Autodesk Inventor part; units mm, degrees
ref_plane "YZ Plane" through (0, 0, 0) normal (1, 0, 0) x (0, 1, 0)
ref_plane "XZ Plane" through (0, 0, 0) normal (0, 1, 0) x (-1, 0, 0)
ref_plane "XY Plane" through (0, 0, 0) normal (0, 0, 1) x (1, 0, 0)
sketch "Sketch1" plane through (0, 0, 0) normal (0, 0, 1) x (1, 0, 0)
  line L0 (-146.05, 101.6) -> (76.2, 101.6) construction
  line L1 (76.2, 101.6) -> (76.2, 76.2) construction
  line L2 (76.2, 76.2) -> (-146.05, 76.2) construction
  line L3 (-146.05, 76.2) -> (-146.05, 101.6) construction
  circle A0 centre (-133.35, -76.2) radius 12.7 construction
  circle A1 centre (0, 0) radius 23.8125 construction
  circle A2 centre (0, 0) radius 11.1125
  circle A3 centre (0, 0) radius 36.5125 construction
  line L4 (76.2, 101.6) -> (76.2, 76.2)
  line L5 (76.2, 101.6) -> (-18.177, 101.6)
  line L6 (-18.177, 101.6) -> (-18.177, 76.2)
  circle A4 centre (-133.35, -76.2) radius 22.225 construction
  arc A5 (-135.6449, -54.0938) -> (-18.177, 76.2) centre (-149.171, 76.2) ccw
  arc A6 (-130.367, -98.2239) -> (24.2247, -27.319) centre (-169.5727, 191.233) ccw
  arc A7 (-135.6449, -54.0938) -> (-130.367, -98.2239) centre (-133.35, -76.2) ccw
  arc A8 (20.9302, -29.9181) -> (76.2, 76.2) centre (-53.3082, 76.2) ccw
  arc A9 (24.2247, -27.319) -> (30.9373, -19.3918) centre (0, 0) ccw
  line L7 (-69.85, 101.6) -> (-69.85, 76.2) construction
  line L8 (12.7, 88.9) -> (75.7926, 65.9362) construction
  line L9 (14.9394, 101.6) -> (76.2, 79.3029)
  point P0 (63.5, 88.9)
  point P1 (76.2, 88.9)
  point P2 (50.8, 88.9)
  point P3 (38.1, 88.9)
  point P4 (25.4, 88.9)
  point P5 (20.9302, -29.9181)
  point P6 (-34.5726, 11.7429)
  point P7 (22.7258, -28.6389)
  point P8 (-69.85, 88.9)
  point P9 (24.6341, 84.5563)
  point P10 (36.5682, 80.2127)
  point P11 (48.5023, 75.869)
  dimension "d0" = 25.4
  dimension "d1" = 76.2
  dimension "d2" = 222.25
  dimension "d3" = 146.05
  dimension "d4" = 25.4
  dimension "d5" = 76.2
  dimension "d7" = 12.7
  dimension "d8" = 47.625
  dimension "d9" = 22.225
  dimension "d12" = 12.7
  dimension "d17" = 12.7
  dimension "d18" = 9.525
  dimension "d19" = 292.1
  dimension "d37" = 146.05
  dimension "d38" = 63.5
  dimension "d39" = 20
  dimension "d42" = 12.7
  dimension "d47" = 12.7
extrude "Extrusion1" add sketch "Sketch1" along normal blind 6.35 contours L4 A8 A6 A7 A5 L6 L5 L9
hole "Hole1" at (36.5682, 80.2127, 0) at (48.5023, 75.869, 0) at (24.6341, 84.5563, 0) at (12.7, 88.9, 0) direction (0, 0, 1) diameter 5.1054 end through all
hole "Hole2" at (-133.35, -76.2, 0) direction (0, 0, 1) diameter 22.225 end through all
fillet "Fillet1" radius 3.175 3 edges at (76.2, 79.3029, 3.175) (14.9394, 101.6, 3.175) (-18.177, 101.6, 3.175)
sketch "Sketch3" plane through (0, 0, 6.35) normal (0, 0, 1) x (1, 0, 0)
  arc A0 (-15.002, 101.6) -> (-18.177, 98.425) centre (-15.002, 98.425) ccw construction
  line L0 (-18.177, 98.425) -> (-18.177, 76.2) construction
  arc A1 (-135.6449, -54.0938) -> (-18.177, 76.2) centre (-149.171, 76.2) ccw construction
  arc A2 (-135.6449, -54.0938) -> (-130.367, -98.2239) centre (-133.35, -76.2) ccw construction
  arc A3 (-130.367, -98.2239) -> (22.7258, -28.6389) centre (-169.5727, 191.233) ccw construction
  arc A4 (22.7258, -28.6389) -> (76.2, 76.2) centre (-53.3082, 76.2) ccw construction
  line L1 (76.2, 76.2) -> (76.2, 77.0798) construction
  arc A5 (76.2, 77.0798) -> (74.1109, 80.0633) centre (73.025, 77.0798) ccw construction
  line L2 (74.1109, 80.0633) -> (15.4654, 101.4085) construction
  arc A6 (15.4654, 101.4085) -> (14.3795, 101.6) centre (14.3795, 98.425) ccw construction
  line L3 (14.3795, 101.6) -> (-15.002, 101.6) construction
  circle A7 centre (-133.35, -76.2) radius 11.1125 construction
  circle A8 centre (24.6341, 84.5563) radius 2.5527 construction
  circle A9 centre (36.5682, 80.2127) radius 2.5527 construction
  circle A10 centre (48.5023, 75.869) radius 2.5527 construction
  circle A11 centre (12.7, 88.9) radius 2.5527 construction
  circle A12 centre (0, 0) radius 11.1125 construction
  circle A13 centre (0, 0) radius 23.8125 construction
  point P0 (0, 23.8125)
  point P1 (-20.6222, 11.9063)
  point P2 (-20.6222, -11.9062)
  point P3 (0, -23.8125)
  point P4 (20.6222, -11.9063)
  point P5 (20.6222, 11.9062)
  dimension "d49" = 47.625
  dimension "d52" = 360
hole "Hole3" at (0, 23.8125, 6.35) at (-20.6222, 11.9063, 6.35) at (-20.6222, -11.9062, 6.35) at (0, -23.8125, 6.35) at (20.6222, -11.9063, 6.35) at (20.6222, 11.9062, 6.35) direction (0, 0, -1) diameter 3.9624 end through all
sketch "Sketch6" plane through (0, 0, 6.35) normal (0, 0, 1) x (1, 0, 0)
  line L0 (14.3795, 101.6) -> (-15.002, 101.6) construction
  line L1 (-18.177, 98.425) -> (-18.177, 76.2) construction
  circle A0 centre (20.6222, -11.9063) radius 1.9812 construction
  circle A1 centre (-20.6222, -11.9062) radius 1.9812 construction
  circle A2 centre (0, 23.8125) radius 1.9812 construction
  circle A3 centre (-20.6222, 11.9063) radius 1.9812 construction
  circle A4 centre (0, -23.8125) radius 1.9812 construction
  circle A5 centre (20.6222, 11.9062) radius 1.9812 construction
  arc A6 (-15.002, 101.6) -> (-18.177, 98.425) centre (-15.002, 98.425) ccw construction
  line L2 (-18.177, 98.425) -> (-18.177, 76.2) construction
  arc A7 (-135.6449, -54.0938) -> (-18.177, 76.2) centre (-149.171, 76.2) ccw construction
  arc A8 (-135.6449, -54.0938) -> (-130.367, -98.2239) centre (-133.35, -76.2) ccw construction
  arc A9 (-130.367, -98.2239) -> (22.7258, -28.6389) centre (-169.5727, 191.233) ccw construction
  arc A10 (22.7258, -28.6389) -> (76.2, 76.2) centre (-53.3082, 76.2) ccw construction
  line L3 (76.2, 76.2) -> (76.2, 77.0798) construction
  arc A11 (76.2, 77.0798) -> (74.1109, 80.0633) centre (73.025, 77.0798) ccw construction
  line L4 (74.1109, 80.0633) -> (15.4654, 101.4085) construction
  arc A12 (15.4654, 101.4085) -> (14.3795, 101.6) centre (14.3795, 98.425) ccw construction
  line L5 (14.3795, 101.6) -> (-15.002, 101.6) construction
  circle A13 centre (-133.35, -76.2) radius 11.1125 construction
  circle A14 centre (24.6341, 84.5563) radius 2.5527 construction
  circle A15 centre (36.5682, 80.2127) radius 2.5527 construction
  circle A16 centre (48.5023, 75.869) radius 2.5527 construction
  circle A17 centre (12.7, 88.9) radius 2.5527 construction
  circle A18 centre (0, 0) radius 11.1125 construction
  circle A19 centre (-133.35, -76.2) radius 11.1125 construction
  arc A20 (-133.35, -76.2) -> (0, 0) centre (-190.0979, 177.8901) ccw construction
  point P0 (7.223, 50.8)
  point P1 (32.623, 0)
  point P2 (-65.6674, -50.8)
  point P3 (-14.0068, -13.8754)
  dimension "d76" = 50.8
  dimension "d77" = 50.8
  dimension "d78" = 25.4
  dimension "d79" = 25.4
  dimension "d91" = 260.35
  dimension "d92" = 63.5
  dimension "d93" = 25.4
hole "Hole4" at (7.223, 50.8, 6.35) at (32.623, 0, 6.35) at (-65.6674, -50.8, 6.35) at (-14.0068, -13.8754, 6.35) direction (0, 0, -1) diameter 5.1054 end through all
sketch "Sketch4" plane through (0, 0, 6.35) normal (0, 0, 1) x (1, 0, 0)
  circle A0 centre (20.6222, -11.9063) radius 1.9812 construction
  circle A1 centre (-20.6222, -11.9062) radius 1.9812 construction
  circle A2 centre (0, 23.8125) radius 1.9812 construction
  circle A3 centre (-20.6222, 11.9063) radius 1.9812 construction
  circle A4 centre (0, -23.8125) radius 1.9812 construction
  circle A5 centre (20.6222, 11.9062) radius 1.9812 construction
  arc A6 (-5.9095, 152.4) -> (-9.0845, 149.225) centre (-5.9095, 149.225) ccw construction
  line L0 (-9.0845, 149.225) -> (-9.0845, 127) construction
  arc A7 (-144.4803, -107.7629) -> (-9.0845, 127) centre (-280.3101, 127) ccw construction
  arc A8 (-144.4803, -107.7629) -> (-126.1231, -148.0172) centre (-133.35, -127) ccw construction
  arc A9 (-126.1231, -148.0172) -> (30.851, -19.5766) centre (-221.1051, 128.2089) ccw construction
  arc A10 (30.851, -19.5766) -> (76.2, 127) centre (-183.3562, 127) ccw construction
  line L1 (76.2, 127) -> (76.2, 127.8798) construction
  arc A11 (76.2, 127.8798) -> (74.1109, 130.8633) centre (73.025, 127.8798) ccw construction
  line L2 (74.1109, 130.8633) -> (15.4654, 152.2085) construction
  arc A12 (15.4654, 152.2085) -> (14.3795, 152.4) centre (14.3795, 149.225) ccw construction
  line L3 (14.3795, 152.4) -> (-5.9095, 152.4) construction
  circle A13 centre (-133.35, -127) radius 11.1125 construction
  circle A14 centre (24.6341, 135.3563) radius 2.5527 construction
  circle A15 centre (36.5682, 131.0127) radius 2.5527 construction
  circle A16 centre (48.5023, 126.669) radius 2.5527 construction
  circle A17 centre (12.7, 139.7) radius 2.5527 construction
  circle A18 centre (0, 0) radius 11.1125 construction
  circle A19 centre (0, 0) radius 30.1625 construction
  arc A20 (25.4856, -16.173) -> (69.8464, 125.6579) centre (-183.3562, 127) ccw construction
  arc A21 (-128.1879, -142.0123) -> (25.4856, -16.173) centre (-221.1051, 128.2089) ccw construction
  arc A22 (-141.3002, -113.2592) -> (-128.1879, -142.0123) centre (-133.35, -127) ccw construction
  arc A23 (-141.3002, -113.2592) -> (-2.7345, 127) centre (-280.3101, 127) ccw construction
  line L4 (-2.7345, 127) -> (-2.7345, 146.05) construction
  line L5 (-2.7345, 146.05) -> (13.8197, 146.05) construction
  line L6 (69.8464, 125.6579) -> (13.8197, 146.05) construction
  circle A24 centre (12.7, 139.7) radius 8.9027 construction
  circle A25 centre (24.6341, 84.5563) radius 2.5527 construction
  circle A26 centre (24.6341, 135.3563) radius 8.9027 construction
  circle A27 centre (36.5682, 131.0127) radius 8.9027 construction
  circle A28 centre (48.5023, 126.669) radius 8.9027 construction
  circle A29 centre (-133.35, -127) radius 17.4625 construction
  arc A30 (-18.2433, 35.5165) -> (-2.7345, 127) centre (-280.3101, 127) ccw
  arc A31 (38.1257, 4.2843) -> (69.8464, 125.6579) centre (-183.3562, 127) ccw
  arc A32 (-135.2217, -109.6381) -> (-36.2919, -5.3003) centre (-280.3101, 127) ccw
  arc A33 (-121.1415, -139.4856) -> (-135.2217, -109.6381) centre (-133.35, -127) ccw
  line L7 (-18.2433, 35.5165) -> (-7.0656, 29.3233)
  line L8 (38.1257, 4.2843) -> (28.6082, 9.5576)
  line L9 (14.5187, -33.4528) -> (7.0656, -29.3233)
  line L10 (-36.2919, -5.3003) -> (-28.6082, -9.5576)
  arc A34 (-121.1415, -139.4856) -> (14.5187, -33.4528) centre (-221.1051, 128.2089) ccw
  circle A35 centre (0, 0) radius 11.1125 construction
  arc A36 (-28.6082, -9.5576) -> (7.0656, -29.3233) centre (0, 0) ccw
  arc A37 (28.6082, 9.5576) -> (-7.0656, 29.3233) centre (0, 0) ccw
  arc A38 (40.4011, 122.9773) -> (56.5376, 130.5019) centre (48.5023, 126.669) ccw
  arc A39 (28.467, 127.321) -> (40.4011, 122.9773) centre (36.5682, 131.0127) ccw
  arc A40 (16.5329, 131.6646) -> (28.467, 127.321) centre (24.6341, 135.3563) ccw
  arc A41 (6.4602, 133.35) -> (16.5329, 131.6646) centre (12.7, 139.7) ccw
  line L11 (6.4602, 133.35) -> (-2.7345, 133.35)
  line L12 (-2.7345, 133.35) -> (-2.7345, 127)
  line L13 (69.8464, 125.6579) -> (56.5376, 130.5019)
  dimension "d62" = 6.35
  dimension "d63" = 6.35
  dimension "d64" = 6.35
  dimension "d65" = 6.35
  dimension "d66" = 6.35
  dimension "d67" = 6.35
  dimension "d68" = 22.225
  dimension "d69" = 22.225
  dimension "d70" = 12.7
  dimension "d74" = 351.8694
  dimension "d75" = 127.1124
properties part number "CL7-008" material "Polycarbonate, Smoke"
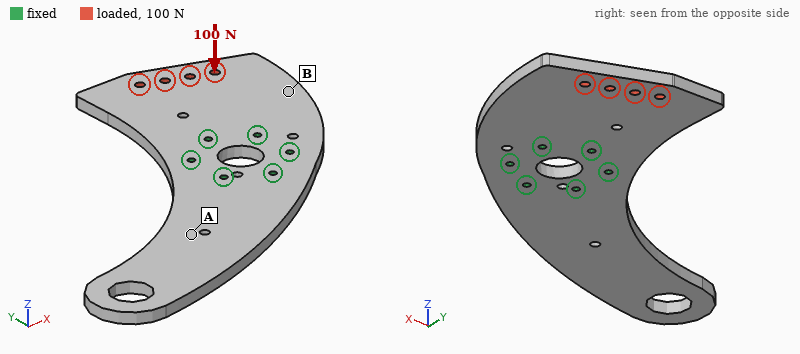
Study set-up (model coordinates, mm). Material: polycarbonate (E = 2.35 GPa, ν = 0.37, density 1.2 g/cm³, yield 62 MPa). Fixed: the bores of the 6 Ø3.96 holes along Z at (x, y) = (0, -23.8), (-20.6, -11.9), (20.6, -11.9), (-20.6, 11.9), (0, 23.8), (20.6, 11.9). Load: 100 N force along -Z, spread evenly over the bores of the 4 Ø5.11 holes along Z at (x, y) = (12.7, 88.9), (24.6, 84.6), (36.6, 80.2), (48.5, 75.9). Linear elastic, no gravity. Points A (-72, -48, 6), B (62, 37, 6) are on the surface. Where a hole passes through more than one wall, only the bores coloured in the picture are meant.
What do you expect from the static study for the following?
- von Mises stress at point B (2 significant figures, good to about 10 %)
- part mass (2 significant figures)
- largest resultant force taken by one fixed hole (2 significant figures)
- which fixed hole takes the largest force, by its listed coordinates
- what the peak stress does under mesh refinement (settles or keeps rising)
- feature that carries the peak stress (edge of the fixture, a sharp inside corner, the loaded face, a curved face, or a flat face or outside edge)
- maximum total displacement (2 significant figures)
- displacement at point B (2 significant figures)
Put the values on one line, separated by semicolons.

4.5 MPa; 130 g; 170 N; (0, 23.8); keeps rising; edge of the fixture; 3.3 mm; 0.91 mm
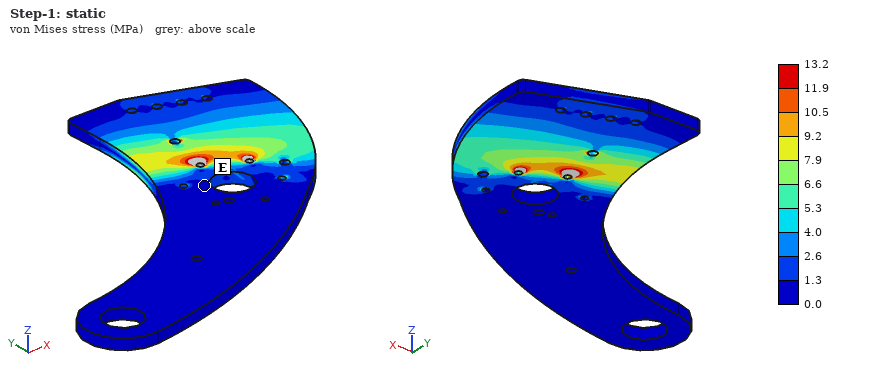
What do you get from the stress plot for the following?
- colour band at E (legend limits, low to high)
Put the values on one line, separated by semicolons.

0.0 to 1.3 MPa
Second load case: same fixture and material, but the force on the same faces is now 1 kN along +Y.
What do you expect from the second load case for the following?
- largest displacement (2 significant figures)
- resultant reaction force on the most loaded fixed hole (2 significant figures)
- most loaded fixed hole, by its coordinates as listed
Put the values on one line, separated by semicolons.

0.21 mm; 590 N; (20.6, 11.9)
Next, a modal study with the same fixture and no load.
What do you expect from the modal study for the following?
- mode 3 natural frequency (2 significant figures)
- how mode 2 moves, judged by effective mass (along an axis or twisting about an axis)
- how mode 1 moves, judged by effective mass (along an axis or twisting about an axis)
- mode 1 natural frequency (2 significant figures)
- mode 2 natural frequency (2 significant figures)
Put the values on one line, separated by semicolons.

340 Hz; along Z; along Z; 77 Hz; 210 Hz
